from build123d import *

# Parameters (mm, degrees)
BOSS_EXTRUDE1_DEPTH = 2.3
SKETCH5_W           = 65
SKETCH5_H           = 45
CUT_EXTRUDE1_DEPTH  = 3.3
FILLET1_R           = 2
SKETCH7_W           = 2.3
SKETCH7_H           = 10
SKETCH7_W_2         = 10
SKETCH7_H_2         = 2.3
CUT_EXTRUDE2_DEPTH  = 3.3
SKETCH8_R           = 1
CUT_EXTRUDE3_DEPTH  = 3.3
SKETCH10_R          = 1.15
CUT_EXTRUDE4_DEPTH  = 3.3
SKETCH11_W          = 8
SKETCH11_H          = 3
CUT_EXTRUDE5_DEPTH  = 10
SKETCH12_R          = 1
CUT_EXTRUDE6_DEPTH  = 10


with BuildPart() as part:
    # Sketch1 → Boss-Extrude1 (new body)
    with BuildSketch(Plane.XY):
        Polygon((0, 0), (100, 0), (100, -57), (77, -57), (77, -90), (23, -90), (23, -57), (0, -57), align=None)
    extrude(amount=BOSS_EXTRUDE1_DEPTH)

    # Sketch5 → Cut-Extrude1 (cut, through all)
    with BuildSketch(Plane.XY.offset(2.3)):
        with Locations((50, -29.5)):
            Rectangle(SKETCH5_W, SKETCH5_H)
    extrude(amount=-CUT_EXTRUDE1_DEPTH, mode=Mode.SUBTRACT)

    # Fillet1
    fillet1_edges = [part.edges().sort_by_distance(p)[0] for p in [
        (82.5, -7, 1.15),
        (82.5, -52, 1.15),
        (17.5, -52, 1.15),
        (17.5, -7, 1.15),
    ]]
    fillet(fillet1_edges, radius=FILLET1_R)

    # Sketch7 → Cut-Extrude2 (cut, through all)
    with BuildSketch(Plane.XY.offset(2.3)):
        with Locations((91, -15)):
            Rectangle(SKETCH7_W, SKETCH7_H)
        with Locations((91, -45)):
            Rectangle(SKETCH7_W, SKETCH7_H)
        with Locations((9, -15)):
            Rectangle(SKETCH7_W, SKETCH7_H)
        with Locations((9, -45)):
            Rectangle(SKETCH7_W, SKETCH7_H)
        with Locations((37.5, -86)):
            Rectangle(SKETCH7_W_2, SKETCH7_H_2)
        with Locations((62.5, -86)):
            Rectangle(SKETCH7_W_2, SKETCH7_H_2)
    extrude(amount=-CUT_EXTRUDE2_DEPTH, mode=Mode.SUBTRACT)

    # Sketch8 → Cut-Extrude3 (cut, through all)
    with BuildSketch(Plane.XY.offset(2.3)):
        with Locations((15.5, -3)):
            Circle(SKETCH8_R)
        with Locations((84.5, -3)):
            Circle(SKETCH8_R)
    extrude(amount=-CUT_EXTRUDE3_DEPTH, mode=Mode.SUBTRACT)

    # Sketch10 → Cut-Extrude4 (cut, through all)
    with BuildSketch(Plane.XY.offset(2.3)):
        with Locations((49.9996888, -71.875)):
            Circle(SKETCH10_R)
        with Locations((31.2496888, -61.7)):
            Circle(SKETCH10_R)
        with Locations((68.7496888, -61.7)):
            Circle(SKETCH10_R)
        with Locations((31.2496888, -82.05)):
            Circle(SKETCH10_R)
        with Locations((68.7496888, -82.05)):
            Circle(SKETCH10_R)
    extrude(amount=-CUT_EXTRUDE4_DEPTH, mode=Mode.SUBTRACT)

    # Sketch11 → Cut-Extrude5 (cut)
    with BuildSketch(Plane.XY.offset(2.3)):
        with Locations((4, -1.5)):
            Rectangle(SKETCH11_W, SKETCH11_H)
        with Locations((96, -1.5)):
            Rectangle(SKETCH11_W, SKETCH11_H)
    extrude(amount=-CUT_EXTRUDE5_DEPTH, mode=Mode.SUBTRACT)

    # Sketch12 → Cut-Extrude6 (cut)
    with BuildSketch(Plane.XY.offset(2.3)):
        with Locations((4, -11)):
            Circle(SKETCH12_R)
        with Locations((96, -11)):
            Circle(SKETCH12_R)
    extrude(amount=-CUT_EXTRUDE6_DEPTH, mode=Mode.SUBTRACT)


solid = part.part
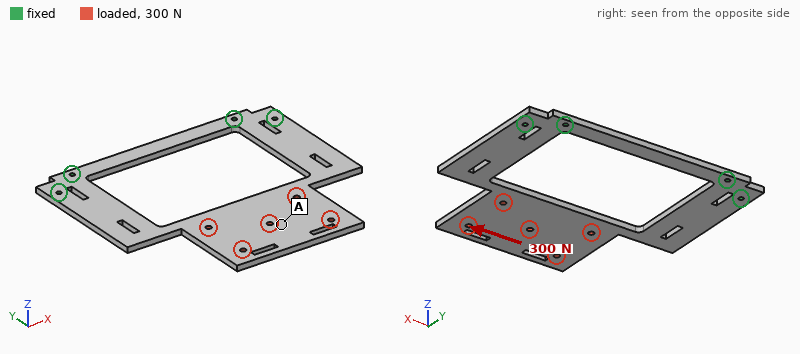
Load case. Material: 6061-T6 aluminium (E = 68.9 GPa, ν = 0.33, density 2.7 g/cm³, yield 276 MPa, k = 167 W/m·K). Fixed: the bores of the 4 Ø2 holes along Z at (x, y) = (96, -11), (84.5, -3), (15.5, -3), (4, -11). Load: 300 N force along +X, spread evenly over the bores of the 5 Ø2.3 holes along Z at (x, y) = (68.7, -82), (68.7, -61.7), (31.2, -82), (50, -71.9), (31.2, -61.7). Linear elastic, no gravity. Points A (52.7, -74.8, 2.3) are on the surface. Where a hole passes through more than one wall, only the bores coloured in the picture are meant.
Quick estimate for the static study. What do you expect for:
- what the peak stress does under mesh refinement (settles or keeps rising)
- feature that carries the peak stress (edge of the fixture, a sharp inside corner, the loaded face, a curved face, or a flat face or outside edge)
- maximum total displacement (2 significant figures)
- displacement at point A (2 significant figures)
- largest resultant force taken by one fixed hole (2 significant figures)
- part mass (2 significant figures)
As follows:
keeps rising
edge of the fixture
70 µm
61 µm
460 N
27 g
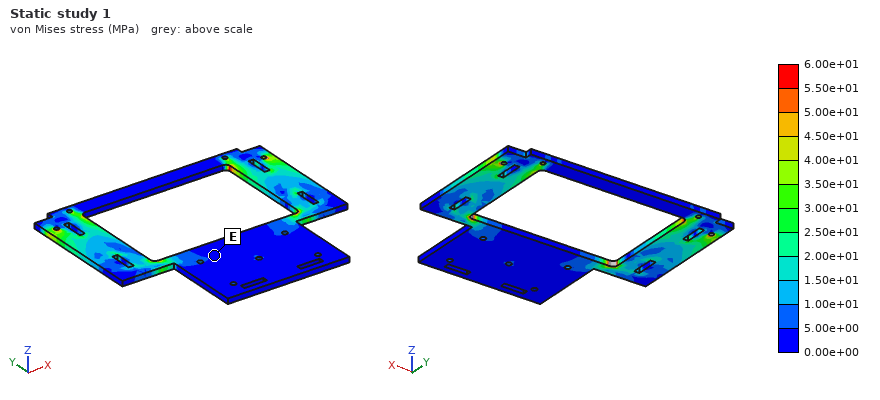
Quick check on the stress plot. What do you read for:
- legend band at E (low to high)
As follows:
0.00e+00 to 5.00e+00 MPa
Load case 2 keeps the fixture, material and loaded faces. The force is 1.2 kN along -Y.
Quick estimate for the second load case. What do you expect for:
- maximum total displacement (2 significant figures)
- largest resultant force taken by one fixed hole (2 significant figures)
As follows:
86 µm
570 N
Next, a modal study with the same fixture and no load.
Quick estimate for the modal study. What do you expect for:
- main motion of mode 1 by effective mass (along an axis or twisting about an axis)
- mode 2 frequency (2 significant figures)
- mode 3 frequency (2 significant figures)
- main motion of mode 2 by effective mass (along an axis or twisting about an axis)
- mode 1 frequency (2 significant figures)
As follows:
along Z
730 Hz
1100 Hz
twisting about Y
210 Hz
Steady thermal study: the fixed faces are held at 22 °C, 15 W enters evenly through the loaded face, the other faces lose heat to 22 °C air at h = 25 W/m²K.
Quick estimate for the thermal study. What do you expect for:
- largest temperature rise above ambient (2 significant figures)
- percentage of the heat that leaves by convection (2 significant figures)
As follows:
64 K
55 %
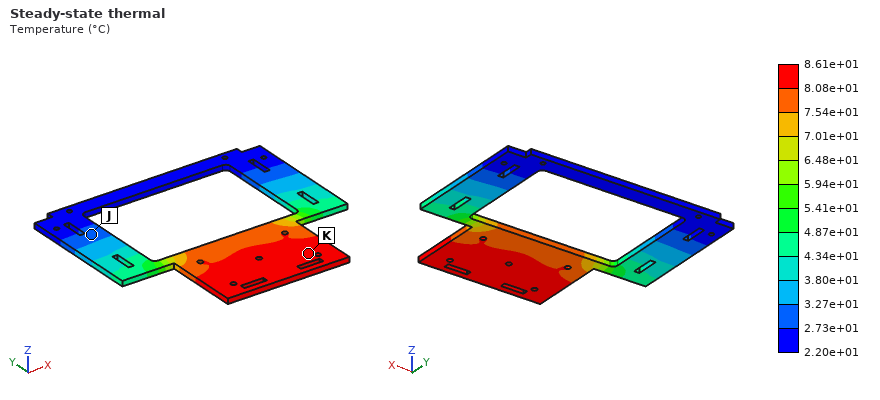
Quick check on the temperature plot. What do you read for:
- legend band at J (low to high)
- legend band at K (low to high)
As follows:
2.73e+01 to 3.27e+01 °C
8.08e+01 to 8.61e+01 °C
